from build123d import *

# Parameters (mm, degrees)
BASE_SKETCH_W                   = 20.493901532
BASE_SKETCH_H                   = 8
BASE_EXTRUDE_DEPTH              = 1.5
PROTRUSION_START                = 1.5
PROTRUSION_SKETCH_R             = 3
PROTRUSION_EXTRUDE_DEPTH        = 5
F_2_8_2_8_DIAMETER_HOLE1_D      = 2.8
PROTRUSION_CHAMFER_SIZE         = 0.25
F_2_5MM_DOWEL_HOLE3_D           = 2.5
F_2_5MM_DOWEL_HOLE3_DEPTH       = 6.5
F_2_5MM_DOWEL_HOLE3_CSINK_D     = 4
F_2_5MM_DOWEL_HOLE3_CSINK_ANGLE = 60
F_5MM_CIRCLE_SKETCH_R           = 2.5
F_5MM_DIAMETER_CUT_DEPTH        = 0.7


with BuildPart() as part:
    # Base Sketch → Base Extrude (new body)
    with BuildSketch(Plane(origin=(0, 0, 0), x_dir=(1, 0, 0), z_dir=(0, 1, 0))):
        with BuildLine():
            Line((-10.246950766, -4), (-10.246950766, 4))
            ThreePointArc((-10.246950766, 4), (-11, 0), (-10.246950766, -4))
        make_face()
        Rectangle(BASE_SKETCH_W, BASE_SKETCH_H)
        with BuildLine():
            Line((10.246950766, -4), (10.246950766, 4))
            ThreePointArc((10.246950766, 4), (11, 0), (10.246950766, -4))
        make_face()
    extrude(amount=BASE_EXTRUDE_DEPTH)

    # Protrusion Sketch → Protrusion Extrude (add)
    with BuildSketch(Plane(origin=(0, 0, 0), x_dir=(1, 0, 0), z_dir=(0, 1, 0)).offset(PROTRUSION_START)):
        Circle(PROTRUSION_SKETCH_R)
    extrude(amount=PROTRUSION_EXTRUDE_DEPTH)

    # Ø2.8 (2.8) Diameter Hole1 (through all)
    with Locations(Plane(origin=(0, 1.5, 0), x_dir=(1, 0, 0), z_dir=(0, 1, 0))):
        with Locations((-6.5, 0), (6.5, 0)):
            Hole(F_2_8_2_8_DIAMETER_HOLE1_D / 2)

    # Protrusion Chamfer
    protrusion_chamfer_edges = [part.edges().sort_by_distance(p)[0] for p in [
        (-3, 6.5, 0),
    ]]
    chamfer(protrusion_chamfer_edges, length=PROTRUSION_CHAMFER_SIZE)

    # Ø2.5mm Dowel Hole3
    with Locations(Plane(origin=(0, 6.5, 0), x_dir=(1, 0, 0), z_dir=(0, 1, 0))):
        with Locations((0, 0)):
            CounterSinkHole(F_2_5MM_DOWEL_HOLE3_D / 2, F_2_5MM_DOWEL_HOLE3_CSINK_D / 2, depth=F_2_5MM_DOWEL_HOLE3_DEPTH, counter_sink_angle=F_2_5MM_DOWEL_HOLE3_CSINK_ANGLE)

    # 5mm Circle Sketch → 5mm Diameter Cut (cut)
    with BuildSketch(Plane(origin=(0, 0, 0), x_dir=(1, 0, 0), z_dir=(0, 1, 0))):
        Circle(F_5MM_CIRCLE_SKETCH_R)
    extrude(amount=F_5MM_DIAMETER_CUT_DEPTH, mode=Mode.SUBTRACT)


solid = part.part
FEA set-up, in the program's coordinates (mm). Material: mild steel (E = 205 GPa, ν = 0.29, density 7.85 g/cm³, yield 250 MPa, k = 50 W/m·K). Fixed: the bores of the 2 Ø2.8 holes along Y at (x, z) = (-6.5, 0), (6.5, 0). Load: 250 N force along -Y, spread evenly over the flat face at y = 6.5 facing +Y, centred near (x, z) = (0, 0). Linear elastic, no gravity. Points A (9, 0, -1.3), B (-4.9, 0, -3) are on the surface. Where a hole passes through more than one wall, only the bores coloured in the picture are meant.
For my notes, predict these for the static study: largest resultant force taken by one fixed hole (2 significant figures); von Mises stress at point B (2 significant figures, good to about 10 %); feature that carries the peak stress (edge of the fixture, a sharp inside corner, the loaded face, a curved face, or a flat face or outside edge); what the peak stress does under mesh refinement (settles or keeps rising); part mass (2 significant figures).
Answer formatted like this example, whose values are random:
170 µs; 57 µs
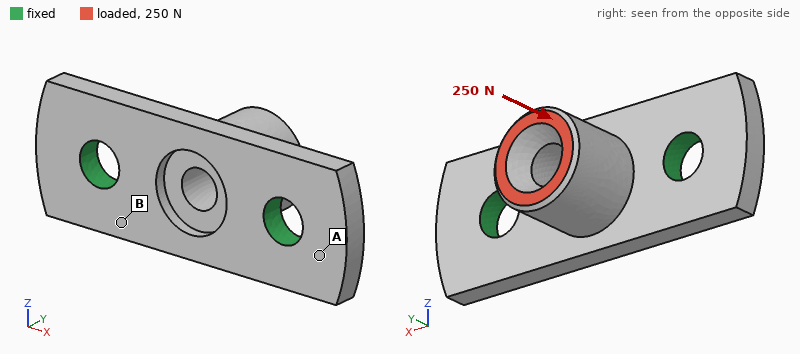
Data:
140 N; 24 MPa; edge of the fixture; keeps rising; 2.6 g
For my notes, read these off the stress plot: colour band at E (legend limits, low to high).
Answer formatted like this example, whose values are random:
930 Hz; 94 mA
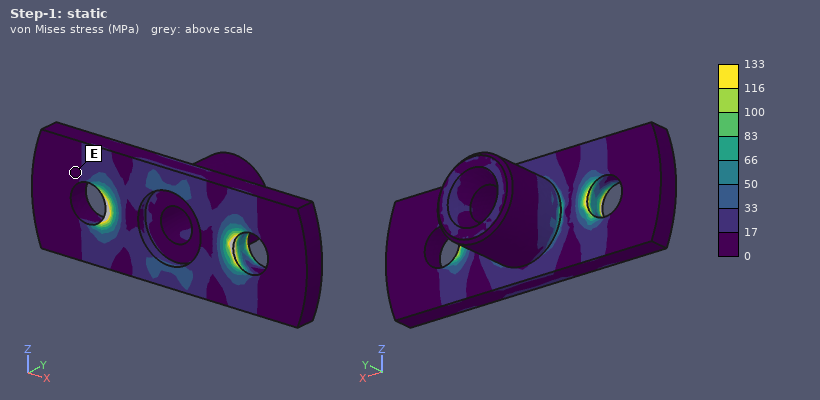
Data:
0 to 17 MPa
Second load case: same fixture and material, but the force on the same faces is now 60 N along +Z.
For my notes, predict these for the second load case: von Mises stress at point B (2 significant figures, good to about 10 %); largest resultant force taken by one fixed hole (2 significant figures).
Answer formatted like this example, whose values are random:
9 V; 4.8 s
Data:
22 MPa; 30 N
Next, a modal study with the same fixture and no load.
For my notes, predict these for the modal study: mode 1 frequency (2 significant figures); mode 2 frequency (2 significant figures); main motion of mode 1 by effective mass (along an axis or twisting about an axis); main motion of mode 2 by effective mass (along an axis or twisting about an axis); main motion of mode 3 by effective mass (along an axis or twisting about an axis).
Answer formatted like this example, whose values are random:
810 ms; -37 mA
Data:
26 kHz; 44 kHz; along Z; along Y; along X
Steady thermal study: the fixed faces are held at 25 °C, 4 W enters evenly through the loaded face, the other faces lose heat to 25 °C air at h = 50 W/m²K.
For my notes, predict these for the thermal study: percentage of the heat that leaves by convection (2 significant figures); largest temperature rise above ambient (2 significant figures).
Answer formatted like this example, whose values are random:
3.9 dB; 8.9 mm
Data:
6.5 %; 33 K
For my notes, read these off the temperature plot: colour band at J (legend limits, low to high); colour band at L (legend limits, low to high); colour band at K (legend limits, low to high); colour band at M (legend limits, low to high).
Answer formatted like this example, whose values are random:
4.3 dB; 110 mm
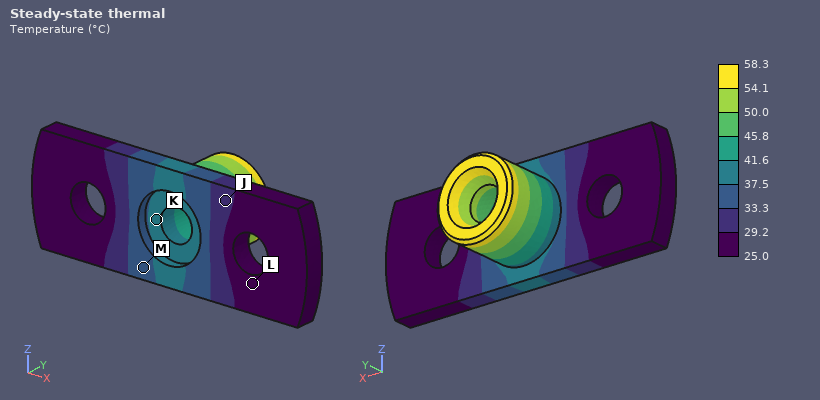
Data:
29.2 to 33.3 °C; 25.0 to 29.2 °C; 37.5 to 41.6 °C; 33.3 to 37.5 °C
